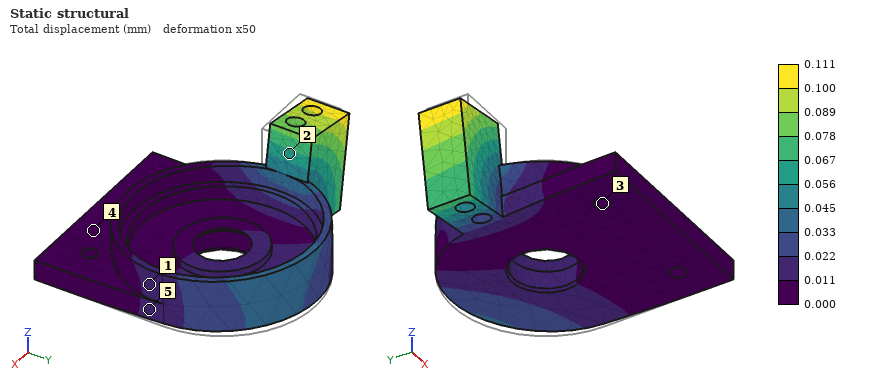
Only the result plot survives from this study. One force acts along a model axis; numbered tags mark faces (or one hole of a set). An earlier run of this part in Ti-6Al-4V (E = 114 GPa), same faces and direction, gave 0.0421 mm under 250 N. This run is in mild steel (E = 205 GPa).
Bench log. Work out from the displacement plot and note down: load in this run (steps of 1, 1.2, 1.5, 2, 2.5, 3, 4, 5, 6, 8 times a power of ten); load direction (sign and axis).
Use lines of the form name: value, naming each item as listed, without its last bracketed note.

load in this run: 1.2 kN
load direction: -X
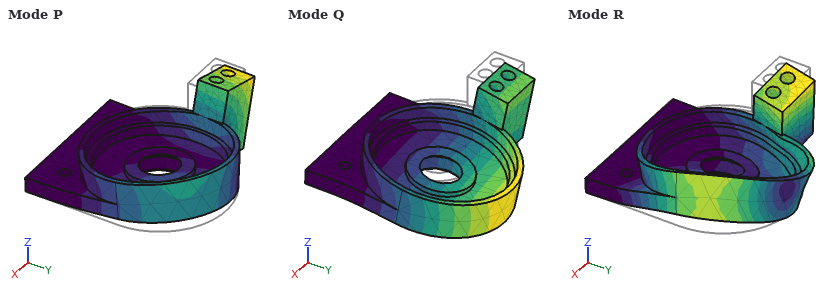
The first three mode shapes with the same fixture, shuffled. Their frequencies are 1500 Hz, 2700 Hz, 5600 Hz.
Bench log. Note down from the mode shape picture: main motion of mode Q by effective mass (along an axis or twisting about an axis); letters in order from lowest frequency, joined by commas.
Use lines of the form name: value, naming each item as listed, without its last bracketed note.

main motion of mode Q by effective mass: along Z
letters in order from lowest frequency, joined by commas: Q, P, R
